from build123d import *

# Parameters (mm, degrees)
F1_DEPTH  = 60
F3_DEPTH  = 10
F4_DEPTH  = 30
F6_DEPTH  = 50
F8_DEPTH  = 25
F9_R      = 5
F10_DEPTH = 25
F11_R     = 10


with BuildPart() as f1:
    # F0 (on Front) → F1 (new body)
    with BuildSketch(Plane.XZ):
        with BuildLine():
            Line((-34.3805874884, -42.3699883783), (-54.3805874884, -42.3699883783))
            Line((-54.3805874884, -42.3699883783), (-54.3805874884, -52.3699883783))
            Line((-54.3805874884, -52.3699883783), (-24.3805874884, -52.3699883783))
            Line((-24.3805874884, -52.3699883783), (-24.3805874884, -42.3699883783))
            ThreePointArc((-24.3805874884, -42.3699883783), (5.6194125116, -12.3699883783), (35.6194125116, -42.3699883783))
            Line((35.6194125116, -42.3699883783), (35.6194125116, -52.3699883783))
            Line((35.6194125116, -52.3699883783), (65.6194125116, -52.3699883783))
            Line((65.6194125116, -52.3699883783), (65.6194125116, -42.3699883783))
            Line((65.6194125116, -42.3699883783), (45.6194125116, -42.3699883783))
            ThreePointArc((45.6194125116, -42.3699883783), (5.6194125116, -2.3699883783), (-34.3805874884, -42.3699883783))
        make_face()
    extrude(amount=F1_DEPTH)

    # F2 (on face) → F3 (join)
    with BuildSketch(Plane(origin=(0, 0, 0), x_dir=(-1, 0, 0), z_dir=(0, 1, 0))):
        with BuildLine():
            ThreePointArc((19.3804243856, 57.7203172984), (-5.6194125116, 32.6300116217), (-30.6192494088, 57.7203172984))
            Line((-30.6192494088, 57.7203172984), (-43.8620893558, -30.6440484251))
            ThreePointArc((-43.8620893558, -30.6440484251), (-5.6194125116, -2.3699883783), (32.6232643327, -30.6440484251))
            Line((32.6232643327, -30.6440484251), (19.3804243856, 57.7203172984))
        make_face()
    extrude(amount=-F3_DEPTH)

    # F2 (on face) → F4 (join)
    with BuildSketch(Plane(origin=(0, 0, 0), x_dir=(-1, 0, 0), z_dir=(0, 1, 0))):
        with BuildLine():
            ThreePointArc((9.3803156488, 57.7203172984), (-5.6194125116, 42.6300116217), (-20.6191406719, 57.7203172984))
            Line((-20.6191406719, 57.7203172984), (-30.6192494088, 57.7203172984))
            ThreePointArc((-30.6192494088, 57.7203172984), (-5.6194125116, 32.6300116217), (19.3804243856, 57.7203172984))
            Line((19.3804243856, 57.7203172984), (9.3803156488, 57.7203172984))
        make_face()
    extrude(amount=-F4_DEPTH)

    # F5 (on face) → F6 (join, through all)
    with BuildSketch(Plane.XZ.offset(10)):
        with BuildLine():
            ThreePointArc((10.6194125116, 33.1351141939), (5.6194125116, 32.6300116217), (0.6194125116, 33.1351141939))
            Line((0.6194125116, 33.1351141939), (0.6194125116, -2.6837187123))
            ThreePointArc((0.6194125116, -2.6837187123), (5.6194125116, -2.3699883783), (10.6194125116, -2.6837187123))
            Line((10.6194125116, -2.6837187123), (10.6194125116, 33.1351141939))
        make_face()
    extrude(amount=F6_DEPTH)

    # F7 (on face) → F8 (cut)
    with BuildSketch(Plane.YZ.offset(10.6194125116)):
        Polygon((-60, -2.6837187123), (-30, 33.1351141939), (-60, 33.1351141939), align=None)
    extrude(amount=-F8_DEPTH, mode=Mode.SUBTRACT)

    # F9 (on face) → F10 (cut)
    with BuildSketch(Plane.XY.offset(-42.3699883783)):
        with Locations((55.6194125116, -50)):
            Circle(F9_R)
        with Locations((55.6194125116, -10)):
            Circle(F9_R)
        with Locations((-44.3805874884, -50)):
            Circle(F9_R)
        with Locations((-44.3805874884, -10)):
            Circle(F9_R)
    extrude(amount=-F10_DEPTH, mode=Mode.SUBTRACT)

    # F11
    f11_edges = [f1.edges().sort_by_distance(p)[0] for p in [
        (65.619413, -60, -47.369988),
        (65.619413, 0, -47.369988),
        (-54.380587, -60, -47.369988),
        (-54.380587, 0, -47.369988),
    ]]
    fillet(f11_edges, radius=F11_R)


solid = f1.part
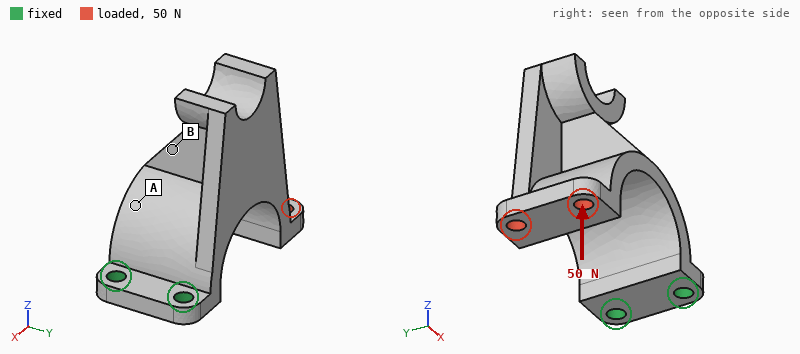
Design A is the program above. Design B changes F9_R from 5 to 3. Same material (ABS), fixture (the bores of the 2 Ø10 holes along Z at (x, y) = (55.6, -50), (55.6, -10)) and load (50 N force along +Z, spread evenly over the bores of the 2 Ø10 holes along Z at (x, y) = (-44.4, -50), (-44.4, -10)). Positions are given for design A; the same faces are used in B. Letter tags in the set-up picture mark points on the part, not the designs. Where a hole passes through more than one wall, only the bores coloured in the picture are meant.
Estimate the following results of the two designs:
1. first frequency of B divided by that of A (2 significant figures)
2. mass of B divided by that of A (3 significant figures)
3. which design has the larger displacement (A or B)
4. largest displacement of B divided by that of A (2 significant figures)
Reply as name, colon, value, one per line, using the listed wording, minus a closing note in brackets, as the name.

first frequency of B divided by that of A: 0.94
mass of B divided by that of A: 1.01
which design has the larger displacement: B
largest displacement of B divided by that of A: 1.1
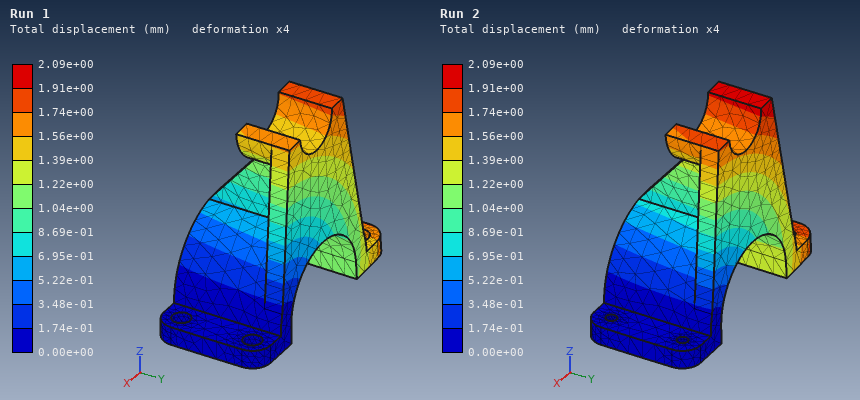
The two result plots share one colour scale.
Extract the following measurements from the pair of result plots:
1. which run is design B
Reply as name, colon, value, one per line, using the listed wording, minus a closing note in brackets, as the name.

which run is design B: Run 2
